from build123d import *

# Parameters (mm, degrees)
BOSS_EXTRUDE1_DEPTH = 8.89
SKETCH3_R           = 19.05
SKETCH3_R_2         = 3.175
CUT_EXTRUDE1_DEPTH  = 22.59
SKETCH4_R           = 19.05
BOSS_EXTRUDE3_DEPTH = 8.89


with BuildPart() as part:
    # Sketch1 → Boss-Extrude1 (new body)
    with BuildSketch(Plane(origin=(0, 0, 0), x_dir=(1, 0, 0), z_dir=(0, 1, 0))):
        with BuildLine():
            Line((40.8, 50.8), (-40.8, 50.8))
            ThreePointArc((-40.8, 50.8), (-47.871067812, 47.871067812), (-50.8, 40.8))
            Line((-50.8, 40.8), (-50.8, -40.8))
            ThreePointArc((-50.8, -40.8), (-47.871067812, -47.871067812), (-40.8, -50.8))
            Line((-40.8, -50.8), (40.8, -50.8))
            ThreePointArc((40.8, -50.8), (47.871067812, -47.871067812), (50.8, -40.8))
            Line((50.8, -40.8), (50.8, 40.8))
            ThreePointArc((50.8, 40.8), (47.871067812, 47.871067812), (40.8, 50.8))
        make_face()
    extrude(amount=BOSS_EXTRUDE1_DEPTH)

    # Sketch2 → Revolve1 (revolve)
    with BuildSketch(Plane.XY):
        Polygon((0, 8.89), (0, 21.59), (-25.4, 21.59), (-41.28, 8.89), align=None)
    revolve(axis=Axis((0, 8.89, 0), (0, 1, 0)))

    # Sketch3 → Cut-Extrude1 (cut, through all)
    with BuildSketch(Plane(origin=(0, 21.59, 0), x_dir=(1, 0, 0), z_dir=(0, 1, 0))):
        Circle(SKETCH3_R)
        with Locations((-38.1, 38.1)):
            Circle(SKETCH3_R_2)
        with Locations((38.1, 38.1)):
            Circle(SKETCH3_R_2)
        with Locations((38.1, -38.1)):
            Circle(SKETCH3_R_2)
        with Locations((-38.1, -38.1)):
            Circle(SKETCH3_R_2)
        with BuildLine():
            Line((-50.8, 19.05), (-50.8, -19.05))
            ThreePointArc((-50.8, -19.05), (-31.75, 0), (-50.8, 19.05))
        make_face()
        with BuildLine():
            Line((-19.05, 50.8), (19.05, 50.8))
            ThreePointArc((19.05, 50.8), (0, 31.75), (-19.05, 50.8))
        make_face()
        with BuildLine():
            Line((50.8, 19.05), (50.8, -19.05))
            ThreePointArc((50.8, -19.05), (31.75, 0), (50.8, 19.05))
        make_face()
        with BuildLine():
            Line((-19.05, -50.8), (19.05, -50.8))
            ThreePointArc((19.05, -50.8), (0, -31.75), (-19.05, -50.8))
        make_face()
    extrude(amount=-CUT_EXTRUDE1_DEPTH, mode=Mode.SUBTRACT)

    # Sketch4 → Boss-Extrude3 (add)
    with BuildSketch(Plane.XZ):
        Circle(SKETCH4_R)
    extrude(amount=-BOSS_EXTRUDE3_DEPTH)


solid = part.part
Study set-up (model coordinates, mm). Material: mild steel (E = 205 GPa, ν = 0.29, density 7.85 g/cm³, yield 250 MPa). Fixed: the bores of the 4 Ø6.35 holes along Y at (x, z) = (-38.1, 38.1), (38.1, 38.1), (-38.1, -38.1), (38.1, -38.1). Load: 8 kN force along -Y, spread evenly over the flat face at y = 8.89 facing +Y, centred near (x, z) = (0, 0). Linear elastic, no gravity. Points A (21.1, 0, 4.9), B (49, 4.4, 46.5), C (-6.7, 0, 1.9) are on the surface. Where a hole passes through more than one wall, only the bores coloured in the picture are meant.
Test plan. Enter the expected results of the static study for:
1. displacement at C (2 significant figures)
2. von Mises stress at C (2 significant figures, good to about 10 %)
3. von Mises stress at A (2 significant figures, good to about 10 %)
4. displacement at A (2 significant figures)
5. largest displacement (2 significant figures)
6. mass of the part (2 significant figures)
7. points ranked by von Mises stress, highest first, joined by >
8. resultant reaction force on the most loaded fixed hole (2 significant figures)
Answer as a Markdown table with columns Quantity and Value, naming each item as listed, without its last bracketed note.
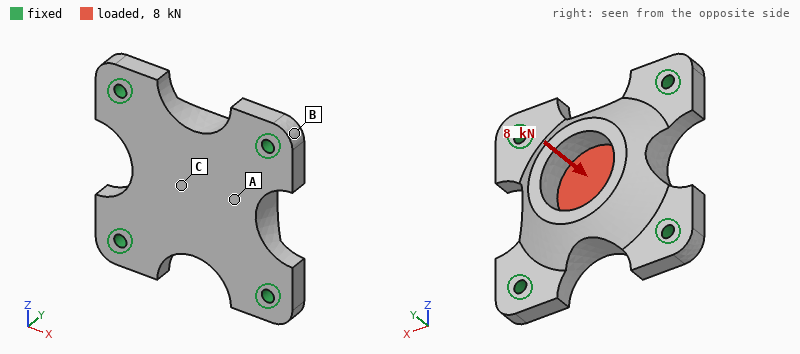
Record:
| Quantity | Value |
|---|---|
| displacement at C | 17 µm |
| von Mises stress at C | 36 MPa |
| von Mises stress at A | 19 MPa |
| displacement at A | 13 µm |
| largest displacement | 18 µm |
| mass of the part | 770 g |
| points ranked by von Mises stress, highest first, joined by > | C > A > B |
| resultant reaction force on the most loaded fixed hole | 2.5 kN |
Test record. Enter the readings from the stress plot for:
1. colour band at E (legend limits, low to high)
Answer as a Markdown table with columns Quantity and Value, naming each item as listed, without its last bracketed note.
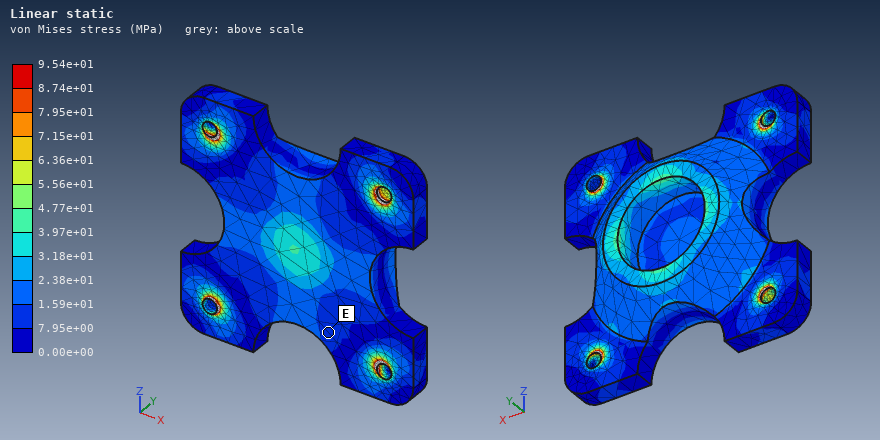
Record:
| Quantity | Value |
|---|---|
| colour band at E | 7.95e+00 to 1.59e+01 MPa |
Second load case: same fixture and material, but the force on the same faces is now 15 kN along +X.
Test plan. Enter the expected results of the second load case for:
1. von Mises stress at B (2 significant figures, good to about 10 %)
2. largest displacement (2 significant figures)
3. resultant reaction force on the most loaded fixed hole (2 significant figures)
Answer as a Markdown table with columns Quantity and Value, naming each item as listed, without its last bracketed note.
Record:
| Quantity | Value |
|---|---|
| von Mises stress at B | 6.1 MPa |
| largest displacement | 6.4 µm |
| resultant reaction force on the most loaded fixed hole | 4.6 kN |
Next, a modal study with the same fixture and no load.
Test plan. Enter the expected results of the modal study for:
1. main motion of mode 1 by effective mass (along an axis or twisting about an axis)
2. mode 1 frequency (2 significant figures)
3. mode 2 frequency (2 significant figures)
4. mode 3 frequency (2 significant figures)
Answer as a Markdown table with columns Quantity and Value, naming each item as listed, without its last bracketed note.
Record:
| Quantity | Value |
|---|---|
| main motion of mode 1 by effective mass | along Y |
| mode 1 frequency | 6200 Hz |
| mode 2 frequency | 10 kHz |
| mode 3 frequency | 10 kHz |
